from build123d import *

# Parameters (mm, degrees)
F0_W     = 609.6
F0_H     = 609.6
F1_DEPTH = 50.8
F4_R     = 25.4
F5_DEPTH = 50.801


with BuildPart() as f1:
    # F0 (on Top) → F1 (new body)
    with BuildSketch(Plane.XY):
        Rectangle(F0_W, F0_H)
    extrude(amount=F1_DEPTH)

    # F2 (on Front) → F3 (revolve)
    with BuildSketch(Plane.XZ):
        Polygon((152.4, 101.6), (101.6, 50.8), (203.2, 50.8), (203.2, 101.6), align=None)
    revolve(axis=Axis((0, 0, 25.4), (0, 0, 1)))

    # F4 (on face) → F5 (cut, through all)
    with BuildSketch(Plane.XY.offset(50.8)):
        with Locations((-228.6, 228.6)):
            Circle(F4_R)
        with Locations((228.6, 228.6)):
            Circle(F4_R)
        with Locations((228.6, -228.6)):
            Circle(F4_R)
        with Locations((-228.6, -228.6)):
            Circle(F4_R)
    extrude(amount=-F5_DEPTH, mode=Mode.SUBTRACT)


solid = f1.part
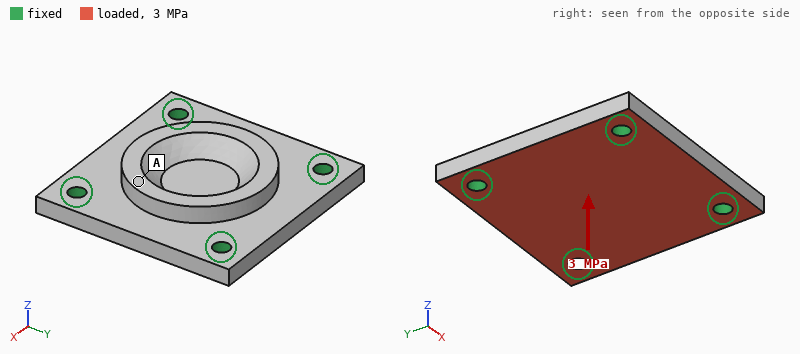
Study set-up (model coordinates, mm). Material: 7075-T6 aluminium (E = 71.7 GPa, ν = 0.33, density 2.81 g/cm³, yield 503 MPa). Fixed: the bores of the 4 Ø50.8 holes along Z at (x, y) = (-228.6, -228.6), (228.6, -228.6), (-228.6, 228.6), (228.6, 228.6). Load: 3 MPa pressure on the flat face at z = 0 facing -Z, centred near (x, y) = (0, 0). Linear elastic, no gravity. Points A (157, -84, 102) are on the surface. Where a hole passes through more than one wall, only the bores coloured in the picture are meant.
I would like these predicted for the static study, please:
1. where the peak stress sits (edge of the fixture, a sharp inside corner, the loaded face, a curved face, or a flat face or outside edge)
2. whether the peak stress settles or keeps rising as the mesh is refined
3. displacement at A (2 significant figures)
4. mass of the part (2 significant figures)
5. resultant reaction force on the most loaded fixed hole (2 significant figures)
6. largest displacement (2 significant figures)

edge of the fixture
keeps rising
0.44 mm
63 kg
280 kN
0.61 mm
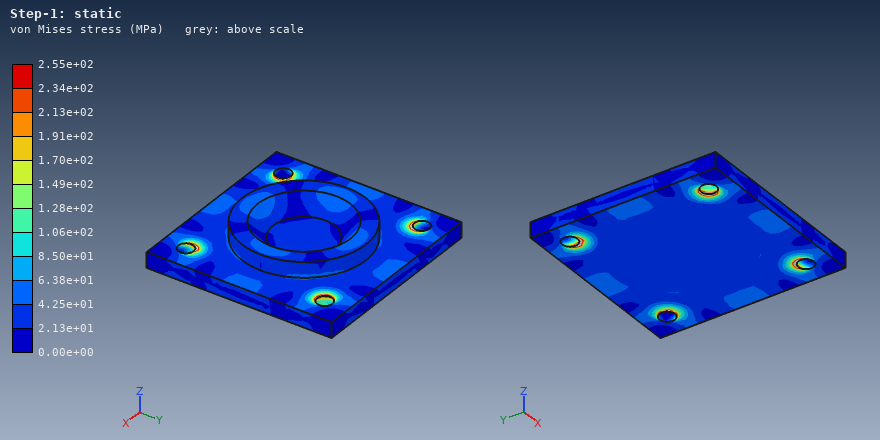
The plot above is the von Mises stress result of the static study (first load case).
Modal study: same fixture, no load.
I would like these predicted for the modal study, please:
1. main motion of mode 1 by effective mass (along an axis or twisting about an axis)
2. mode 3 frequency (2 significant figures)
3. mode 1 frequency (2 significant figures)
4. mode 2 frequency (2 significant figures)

along Z
1400 Hz
950 Hz
1400 Hz
